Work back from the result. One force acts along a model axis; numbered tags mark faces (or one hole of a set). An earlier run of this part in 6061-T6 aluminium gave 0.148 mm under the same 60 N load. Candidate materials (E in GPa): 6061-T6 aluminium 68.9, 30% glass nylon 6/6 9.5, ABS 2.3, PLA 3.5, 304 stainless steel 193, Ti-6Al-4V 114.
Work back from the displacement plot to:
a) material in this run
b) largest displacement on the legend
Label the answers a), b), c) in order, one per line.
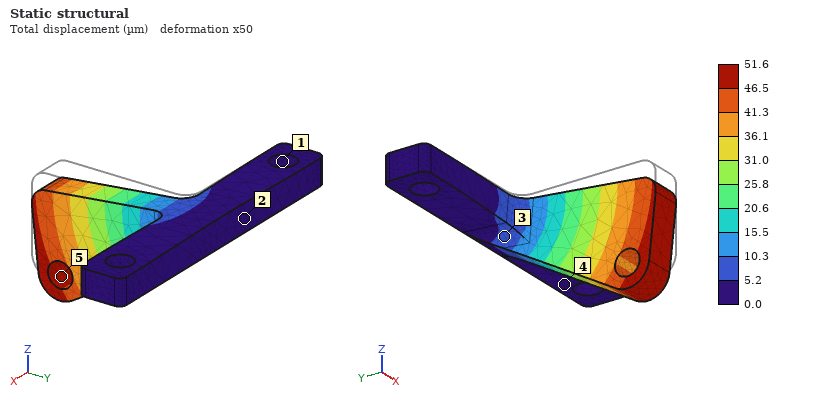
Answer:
a) 304 stainless steel
b) 51.6 µm
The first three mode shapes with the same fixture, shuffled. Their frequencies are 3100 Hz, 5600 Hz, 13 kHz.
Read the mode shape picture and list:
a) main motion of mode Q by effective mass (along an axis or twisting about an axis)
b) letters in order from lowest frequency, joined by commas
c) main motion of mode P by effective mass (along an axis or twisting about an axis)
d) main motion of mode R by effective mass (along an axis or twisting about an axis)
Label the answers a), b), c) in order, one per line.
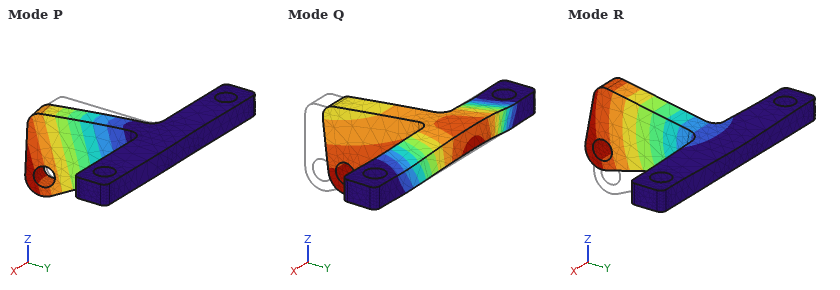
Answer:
a) along Y
b) R, P, Q
c) along X
d) along Z
